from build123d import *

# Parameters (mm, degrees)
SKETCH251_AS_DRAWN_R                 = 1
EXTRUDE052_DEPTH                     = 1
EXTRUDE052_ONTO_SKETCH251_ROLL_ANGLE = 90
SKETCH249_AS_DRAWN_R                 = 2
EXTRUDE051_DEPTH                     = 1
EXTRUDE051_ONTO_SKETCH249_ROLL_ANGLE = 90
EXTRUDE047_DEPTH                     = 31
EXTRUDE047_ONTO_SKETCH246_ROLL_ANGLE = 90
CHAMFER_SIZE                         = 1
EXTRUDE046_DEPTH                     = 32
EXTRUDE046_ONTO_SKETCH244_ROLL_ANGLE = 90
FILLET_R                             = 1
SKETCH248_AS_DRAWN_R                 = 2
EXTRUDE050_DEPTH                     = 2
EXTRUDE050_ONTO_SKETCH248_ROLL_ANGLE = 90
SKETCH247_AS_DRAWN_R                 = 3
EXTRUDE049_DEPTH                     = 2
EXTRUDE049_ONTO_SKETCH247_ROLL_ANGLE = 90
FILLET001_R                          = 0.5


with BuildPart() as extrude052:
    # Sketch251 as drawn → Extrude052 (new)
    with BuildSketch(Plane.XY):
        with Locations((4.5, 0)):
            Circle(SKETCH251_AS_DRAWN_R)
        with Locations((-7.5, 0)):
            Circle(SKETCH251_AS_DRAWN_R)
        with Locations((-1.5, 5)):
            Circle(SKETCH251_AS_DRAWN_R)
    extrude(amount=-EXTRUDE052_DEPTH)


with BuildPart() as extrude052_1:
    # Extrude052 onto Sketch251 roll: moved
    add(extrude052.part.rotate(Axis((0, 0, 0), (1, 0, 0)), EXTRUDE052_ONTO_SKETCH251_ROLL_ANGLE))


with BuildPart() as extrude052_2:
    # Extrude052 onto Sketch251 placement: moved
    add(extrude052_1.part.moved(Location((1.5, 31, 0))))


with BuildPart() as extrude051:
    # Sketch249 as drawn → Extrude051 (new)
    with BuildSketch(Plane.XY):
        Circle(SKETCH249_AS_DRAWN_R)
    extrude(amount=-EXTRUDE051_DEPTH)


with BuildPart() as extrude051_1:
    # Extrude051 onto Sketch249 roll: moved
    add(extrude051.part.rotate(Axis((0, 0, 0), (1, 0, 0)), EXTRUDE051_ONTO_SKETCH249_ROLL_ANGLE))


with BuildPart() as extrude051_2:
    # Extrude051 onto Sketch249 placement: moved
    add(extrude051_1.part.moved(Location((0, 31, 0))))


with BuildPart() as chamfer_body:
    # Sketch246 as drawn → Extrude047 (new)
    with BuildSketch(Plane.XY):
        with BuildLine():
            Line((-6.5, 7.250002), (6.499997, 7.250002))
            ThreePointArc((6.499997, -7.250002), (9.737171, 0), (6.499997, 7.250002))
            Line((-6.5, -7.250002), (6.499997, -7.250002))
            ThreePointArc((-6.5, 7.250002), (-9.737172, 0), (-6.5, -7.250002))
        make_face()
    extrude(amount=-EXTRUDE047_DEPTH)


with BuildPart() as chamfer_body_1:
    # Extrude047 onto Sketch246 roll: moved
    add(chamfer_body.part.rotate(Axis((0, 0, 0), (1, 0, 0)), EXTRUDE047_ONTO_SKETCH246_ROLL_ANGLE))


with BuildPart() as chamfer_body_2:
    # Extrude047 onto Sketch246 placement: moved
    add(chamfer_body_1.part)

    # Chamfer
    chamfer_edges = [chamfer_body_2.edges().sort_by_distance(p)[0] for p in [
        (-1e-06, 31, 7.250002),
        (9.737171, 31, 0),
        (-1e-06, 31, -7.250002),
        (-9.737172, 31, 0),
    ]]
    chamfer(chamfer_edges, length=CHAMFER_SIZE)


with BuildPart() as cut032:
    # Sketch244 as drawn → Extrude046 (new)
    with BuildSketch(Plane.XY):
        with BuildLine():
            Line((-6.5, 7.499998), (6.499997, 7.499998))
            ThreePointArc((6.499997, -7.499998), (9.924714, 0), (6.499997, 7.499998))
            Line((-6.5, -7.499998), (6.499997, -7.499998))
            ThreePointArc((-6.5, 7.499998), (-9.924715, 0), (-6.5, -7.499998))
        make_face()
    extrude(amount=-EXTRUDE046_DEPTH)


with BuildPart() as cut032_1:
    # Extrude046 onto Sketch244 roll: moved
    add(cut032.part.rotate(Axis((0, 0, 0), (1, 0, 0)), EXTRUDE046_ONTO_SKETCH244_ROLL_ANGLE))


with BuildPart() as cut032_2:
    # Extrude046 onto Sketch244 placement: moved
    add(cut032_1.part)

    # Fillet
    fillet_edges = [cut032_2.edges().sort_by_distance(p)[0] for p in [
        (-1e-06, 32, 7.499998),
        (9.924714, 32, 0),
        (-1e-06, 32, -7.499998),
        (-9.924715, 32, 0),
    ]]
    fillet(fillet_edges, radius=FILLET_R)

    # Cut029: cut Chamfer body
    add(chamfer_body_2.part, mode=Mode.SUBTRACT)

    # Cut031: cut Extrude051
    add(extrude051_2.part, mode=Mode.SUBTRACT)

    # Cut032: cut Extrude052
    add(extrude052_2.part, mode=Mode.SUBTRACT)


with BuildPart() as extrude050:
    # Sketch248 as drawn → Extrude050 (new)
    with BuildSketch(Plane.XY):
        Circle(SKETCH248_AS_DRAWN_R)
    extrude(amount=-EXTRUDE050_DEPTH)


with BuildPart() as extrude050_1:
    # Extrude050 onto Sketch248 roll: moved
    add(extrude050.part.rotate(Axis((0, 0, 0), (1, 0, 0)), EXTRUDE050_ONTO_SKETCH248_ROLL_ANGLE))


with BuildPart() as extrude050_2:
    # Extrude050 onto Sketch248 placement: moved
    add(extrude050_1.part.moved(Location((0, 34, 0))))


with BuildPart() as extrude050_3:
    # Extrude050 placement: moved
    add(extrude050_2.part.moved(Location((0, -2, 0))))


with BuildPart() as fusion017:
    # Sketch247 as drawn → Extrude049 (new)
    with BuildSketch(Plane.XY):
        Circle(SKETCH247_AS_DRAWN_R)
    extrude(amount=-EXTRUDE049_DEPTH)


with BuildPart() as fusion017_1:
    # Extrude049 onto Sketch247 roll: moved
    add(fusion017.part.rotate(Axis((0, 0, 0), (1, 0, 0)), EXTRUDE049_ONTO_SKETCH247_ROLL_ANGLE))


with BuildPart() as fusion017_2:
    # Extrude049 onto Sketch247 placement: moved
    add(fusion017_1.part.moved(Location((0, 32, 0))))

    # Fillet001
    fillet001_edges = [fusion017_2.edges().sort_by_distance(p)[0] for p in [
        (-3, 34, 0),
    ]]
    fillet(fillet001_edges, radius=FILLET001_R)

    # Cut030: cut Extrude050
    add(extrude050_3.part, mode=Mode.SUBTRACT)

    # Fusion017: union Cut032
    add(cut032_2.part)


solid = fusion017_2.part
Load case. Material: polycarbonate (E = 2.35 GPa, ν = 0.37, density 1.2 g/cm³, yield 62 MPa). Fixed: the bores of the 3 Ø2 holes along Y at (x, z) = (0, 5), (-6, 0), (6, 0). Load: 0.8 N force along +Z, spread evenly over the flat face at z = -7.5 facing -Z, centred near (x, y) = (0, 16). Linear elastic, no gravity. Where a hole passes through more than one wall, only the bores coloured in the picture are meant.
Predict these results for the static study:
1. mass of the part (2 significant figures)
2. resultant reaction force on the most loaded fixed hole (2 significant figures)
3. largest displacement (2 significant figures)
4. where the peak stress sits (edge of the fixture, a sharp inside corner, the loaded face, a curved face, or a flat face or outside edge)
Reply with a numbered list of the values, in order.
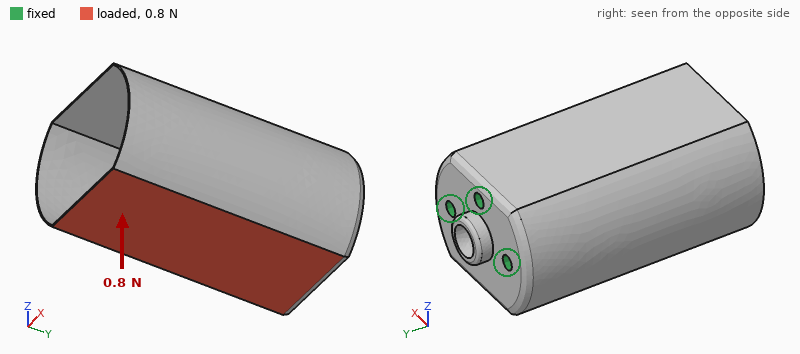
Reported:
1. 0.82 g
2. 1.0 N
3. 0.48 mm
4. the loaded face
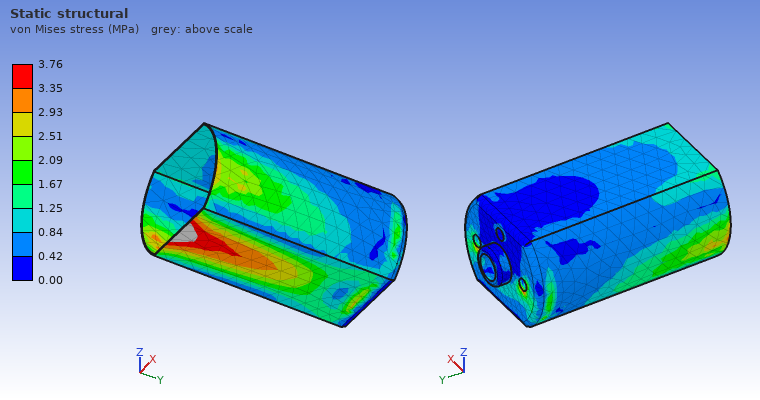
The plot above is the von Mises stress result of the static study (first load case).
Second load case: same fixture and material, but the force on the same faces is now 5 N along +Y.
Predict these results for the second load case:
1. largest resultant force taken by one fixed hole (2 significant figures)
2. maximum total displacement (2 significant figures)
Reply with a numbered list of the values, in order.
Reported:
1. 4.4 N
2. 0.43 mm
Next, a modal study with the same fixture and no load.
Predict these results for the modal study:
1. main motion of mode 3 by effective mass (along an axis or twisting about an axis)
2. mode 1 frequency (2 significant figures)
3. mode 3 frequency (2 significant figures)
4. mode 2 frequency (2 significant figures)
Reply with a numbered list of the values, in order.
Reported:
1. along Z
2. 610 Hz
3. 950 Hz
4. 730 Hz
